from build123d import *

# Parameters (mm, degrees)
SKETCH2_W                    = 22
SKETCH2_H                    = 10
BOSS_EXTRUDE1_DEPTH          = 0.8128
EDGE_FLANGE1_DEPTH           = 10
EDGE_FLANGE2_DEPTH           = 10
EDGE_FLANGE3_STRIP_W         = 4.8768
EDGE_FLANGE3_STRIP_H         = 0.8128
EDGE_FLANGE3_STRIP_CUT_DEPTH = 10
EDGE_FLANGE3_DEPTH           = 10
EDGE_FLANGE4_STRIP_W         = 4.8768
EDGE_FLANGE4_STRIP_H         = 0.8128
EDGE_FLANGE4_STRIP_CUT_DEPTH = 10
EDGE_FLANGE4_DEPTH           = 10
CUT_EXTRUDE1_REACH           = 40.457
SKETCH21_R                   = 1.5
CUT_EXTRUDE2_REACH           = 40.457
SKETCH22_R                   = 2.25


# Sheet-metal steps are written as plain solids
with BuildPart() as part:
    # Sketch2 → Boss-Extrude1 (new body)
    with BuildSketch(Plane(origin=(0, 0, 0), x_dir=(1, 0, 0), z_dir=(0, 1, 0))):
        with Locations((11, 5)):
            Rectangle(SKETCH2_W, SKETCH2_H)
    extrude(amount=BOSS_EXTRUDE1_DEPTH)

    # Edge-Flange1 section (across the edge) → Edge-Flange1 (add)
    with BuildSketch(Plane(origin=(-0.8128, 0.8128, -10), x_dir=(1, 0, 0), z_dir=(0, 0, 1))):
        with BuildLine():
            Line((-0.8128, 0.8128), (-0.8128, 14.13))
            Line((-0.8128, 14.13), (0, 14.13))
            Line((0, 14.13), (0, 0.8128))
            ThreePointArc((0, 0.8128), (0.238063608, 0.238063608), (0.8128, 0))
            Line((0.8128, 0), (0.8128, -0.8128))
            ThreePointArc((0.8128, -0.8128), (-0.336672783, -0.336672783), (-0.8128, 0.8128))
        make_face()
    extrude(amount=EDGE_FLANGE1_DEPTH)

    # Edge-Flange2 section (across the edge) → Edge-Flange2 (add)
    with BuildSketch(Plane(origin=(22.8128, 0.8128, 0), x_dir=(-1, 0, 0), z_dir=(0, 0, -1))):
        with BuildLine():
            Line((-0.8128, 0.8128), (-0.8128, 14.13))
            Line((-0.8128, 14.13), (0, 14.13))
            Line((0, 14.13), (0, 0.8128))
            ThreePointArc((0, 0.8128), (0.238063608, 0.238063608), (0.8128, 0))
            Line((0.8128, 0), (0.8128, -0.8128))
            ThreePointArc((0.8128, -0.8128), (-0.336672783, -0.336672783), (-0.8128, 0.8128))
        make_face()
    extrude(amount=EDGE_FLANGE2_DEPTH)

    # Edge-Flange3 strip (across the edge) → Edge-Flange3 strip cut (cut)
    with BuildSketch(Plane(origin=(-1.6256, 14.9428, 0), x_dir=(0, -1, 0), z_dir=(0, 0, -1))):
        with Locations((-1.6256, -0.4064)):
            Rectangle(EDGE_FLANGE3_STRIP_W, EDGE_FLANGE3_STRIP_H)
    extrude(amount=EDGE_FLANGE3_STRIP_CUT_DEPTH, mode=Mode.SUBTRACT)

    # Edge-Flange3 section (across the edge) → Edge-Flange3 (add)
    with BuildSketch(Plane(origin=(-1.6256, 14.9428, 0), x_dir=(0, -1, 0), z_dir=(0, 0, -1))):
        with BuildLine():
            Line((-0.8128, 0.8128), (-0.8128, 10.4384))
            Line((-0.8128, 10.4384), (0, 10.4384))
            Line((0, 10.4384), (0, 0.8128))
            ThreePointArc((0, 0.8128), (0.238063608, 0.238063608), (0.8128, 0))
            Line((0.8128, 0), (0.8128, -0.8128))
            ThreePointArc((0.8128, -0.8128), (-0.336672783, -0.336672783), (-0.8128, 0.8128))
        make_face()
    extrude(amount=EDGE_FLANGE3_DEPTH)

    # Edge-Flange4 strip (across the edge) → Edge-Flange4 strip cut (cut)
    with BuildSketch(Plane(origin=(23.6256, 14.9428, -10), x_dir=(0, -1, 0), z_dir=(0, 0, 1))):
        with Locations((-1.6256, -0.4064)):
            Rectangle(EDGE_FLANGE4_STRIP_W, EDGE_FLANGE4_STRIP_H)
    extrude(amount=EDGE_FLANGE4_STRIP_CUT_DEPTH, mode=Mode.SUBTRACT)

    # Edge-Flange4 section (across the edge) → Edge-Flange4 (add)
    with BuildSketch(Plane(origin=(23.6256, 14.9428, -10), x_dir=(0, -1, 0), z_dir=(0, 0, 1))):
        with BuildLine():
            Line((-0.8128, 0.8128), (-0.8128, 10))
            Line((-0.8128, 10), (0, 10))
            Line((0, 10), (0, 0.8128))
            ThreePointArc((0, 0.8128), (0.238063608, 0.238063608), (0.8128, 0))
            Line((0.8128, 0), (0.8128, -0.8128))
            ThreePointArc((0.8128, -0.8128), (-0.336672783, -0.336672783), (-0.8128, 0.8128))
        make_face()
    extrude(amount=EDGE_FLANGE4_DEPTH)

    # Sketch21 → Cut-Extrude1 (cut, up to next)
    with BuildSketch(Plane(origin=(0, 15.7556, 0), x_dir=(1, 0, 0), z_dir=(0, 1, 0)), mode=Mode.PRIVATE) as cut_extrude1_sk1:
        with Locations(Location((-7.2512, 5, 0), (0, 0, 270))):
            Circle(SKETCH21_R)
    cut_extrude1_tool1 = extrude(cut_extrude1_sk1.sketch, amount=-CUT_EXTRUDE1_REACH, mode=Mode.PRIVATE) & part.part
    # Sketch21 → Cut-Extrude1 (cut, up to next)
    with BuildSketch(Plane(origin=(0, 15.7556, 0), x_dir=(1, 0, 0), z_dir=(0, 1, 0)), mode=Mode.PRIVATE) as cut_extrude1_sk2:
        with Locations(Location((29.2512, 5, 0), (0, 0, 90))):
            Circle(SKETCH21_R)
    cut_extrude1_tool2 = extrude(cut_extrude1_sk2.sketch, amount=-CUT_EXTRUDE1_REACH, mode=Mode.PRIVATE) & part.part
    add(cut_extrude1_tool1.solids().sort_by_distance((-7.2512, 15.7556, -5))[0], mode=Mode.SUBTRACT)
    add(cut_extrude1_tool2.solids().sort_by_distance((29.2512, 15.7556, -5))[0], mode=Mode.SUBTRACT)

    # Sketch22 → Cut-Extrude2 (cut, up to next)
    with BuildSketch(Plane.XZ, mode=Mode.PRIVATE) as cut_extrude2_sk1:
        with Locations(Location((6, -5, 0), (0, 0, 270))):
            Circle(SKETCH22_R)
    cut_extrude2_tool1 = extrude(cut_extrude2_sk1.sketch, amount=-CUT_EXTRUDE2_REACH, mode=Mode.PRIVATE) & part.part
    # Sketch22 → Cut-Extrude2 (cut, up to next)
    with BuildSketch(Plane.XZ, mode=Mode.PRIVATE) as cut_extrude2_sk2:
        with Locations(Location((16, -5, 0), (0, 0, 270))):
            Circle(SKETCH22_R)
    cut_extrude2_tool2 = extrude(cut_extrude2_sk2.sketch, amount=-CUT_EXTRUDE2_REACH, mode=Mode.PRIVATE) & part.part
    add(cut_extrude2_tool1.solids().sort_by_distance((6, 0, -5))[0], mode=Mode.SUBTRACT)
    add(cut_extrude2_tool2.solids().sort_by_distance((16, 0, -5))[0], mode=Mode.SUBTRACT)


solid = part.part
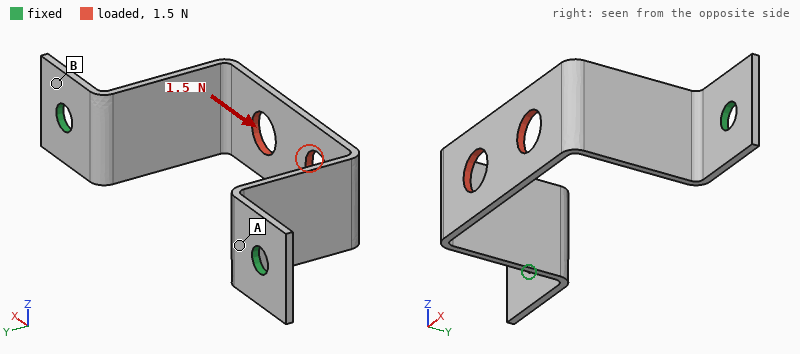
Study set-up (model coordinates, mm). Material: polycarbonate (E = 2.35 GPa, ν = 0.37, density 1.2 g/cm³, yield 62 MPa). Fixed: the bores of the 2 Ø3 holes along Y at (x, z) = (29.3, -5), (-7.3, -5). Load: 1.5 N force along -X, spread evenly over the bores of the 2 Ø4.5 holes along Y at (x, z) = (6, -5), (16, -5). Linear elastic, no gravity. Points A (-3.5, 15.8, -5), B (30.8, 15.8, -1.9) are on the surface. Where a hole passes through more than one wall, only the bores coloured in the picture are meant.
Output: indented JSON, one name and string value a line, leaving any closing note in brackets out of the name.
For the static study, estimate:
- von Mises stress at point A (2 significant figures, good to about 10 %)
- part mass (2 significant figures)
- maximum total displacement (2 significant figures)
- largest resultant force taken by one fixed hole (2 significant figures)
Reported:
{
  "von Mises stress at point A": "3.8 MPa",
  "part mass": "0.67 g",
  "maximum total displacement": "0.45 mm",
  "largest resultant force taken by one fixed hole": "0.88 N"
}
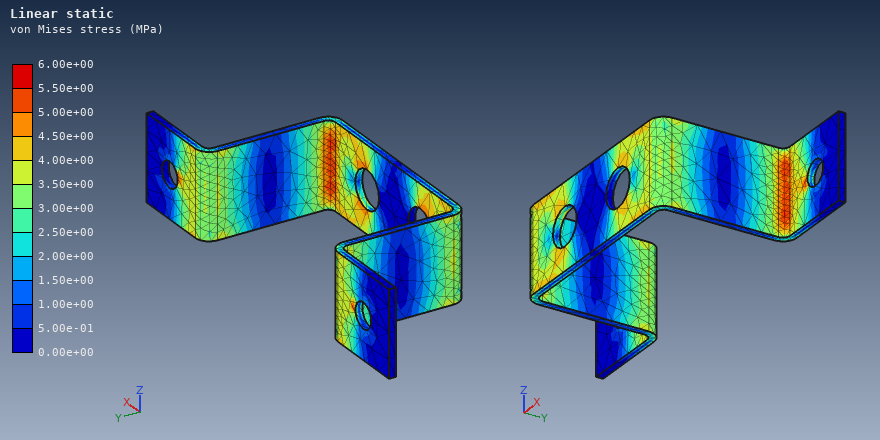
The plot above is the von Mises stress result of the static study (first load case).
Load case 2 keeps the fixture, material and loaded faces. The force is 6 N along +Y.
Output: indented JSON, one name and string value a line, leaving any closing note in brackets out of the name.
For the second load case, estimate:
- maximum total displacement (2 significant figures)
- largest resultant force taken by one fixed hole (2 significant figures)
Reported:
{
  "maximum total displacement": "0.54 mm",
  "largest resultant force taken by one fixed hole": "3.3 N"
}
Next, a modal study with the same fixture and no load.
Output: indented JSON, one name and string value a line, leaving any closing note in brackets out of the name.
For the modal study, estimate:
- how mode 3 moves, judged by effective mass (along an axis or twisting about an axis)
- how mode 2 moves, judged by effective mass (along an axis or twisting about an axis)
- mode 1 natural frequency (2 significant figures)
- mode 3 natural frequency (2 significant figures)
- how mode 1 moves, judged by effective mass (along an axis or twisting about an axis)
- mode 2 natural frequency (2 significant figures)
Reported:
{
  "how mode 3 moves, judged by effective mass": "twisting about Y",
  "how mode 2 moves, judged by effective mass": "along Z",
  "mode 1 natural frequency": "530 Hz",
  "mode 3 natural frequency": "880 Hz",
  "how mode 1 moves, judged by effective mass": "along X",
  "mode 2 natural frequency": "580 Hz"
}
